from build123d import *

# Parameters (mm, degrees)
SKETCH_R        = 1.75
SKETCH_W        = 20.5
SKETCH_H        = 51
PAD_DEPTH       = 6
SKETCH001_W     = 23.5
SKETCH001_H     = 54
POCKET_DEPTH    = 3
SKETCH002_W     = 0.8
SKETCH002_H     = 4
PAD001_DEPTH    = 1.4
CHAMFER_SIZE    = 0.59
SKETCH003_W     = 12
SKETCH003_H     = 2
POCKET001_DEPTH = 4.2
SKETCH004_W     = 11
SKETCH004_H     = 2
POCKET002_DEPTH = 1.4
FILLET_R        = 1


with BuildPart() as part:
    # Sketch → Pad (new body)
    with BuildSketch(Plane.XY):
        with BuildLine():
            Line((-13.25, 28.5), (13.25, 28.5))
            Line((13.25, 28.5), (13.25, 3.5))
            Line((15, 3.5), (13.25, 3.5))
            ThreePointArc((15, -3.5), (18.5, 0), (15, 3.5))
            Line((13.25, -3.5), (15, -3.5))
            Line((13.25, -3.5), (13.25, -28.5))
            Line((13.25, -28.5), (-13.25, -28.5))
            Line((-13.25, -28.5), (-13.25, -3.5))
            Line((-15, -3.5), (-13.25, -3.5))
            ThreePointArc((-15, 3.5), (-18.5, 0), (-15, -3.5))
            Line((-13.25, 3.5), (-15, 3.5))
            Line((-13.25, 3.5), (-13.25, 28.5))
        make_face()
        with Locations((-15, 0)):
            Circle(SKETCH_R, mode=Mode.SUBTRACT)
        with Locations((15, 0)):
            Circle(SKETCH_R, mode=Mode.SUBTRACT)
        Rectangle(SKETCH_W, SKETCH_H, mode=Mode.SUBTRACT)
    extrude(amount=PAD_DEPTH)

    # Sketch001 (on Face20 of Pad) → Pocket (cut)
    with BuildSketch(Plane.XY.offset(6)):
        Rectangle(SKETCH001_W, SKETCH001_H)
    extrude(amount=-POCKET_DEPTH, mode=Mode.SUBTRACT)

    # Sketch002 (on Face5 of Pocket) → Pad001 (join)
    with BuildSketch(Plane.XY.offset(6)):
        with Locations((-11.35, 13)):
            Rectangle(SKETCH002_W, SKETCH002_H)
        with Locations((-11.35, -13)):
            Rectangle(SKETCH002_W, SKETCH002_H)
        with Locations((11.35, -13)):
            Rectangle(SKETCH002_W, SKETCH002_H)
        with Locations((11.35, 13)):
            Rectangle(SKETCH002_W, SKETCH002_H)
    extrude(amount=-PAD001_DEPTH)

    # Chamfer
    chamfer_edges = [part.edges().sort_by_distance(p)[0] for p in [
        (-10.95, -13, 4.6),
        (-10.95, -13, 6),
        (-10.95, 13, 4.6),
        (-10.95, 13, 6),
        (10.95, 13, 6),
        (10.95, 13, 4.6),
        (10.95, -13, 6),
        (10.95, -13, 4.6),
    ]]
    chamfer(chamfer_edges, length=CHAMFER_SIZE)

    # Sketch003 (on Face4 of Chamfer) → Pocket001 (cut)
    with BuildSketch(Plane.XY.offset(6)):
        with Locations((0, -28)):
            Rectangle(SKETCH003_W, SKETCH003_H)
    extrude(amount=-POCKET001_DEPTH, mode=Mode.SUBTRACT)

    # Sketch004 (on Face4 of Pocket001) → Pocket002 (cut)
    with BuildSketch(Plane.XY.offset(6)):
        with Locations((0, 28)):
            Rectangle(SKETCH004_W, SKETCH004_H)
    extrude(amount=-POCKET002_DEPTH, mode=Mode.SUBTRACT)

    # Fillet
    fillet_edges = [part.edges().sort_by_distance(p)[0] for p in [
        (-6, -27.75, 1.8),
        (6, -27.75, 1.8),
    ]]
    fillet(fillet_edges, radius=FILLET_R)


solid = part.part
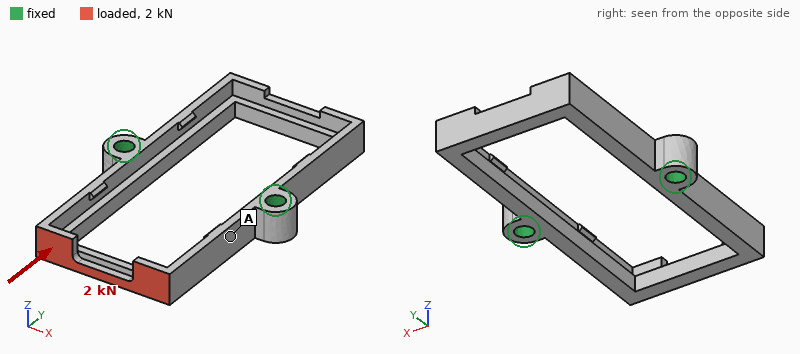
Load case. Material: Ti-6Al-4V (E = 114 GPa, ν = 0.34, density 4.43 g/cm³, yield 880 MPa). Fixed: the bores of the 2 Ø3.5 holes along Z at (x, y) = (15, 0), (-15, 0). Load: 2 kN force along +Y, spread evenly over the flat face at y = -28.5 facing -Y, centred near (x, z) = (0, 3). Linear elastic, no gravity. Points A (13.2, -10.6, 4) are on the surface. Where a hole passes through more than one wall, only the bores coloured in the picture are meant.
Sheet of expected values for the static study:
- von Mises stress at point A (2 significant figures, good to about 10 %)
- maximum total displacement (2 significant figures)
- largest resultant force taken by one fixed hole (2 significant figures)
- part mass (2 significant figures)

75 MPa
0.17 mm
1.0 kN
10 g
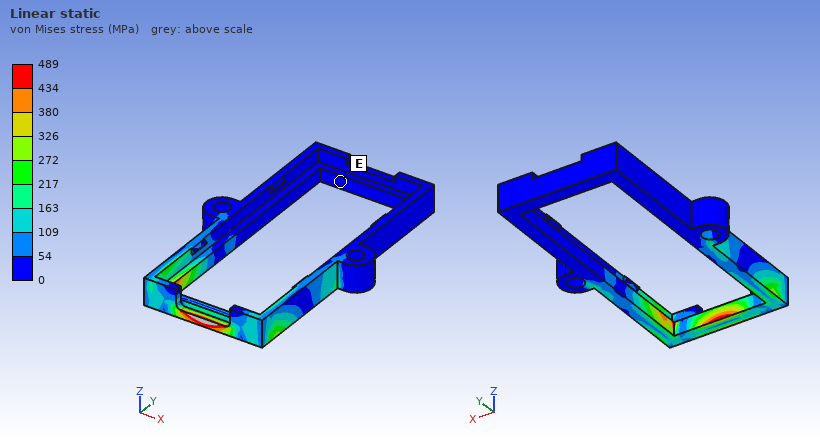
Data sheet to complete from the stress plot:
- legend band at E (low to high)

0 to 54 MPa
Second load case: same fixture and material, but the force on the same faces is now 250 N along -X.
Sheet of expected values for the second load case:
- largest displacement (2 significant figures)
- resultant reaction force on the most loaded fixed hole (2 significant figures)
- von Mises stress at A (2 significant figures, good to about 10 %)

0.28 mm
180 N
97 MPa
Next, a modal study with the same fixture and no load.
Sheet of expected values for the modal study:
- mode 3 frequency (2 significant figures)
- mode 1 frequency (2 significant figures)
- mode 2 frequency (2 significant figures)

3900 Hz
3300 Hz
3400 Hz
